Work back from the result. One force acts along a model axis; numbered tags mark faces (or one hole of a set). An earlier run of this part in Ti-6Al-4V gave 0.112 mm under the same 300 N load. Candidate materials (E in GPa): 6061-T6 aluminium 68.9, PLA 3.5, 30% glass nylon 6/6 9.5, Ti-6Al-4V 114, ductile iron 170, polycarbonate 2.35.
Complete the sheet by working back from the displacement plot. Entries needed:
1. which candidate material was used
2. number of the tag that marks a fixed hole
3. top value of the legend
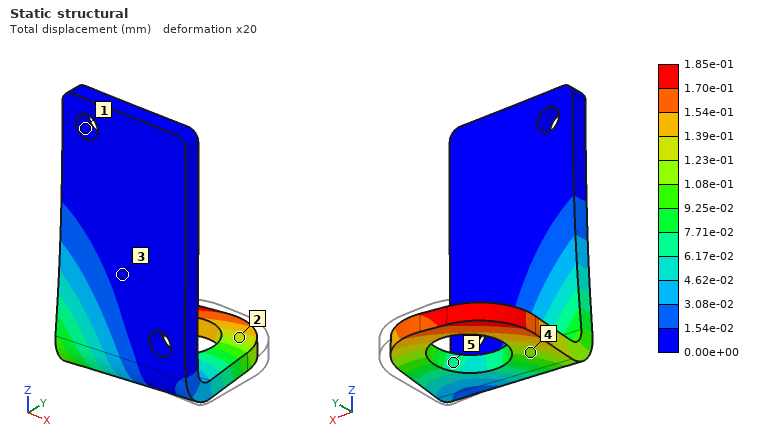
6061-T6 aluminium
1
1.85e-01 mm
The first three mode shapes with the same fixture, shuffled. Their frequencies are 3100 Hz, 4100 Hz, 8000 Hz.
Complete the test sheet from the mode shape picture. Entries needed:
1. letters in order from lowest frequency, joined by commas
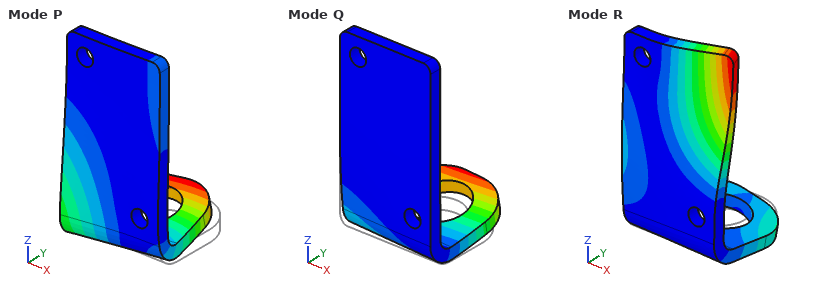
Q, P, R
